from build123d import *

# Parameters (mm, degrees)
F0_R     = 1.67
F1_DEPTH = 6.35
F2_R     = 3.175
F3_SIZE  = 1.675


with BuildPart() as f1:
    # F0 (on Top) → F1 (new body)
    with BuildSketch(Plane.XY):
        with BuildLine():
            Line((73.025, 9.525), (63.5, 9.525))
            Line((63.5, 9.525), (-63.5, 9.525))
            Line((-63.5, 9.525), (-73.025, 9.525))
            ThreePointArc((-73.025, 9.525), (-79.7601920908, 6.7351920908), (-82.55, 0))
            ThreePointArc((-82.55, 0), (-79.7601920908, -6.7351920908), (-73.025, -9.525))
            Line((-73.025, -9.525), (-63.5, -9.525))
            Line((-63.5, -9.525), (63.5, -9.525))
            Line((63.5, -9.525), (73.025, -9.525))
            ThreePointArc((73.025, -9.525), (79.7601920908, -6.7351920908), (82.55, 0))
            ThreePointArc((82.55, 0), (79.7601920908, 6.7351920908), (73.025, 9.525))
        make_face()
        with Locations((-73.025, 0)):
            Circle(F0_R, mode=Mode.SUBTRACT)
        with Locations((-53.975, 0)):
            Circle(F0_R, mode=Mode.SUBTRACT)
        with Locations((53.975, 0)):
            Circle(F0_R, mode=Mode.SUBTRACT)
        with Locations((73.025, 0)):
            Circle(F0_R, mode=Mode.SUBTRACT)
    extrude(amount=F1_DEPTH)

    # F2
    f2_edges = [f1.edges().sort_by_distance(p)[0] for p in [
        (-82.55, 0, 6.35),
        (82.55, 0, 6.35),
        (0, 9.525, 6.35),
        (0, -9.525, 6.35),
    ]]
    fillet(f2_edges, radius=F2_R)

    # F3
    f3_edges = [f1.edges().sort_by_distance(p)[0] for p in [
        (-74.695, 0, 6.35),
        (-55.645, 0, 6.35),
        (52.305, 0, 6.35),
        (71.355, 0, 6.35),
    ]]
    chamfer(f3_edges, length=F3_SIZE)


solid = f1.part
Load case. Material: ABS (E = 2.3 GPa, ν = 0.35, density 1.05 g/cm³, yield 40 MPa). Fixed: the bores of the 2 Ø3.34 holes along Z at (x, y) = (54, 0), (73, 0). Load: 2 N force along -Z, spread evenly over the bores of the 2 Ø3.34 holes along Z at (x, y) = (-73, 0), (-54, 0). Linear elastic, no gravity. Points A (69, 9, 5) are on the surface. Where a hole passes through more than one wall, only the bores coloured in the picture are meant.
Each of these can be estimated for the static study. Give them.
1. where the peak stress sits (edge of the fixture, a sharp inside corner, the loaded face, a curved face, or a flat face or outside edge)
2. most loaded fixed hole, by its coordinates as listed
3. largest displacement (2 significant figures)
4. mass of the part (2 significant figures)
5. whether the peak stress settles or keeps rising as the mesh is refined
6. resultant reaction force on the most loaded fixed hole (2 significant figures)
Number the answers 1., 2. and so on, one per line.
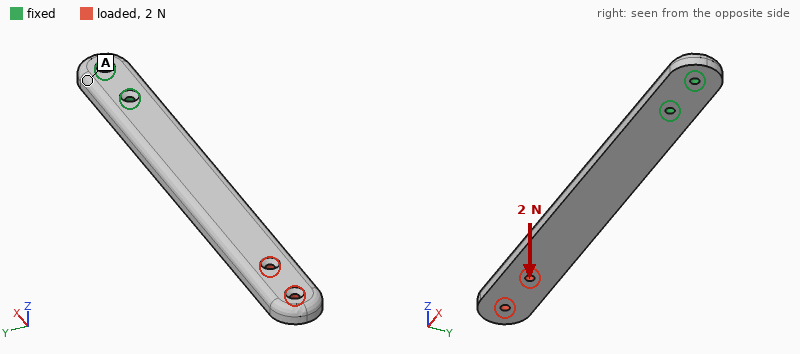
1. edge of the fixture
2. (54, 0)
3. 1.6 mm
4. 19 g
5. keeps rising
6. 8.4 N
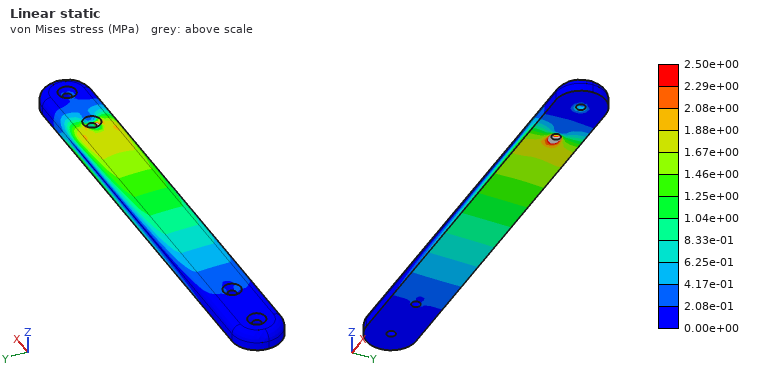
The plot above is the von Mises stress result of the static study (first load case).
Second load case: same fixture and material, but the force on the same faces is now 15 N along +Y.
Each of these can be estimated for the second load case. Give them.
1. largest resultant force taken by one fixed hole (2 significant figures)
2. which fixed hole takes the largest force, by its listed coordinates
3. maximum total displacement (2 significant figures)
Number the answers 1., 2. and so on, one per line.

1. 88 N
2. (54, 0)
3. 1.6 mm
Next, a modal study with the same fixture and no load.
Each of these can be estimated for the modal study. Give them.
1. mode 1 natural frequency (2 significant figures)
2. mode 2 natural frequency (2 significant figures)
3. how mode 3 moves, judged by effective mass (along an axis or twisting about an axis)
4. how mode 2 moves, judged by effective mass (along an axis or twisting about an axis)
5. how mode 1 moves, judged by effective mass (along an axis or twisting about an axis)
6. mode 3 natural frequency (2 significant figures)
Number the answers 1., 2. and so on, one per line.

1. 81 Hz
2. 220 Hz
3. along Z
4. along Y
5. along Z
6. 500 Hz
